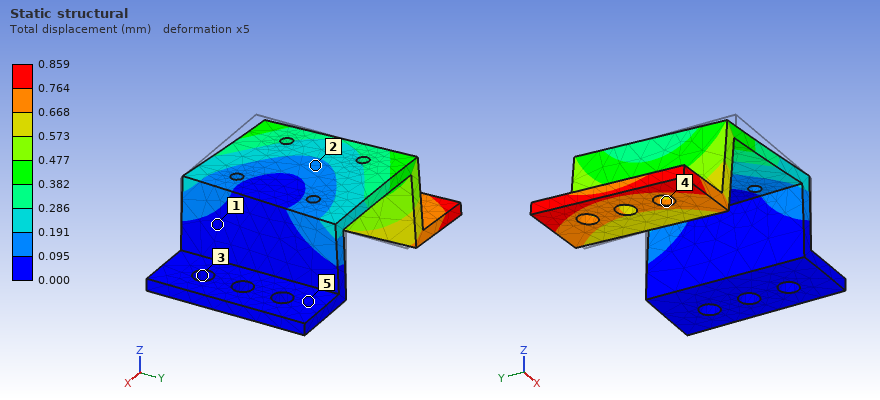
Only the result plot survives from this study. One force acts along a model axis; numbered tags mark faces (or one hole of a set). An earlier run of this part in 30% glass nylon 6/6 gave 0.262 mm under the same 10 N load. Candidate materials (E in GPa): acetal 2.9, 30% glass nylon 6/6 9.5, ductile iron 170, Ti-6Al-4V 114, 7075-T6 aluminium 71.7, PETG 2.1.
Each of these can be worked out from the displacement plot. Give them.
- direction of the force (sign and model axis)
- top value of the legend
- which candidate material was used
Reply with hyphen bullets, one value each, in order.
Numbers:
- +Y
- 0.859 mm
- acetal
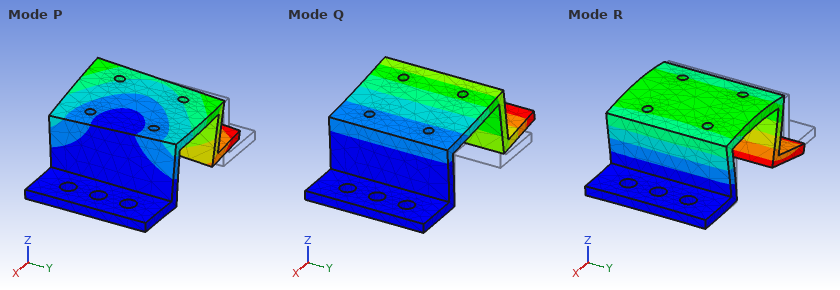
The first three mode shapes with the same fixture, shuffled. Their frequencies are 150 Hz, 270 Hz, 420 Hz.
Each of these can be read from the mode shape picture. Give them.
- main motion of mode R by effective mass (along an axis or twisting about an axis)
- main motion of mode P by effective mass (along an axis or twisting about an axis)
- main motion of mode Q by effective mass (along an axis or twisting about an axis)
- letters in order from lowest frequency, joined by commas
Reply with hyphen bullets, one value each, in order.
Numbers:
- along X
- along Y
- along Z
- Q, P, R
